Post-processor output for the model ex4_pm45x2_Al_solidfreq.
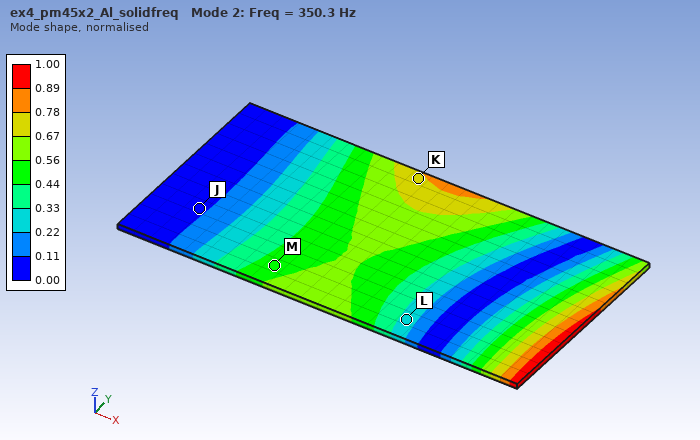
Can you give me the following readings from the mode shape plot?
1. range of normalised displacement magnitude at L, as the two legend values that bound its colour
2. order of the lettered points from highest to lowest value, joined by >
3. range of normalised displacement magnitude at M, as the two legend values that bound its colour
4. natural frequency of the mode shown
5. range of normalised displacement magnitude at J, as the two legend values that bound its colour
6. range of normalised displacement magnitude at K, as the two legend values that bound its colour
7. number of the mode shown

0.22 to 0.33
K > M > L > J
0.44 to 0.56
350.3 Hz
0.00 to 0.11
0.67 to 0.78
2
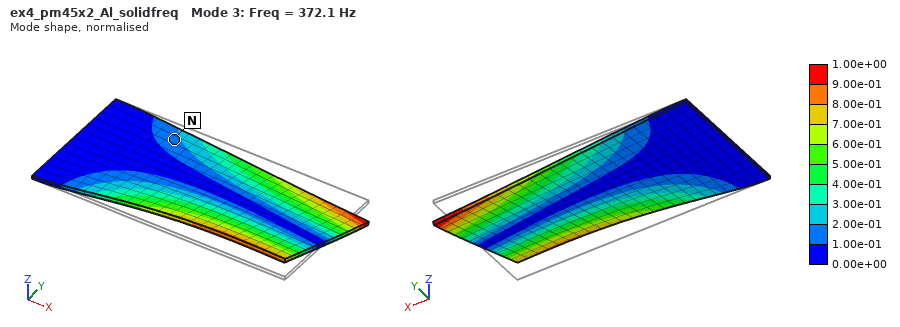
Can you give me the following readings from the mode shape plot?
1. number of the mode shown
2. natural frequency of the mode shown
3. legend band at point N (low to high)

3
372.1 Hz
1.00e-01 to 2.00e-01
